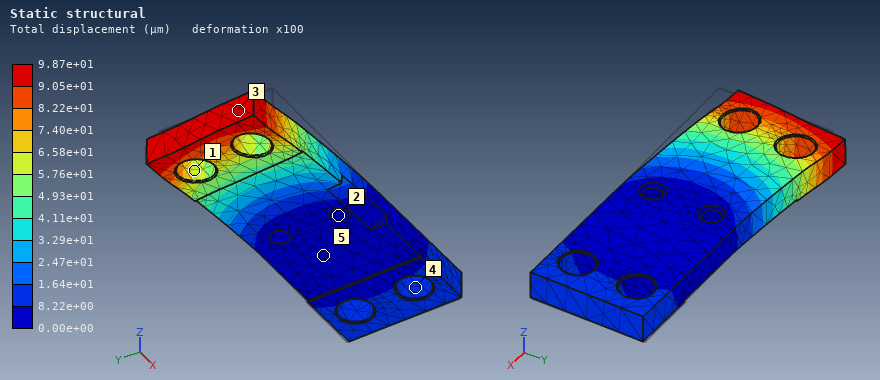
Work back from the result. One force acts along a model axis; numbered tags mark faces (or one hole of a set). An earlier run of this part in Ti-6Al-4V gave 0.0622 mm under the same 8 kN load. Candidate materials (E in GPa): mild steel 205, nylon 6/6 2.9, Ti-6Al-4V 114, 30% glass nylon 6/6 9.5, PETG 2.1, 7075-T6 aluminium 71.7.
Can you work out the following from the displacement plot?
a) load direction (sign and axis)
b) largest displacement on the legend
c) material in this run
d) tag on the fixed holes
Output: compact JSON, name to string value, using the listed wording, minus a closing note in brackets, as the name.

{"load direction": "+Y", "largest displacement on the legend": "9.87e+01 µm", "material in this run": "7075-T6 aluminium", "tag on the fixed holes": "2"}
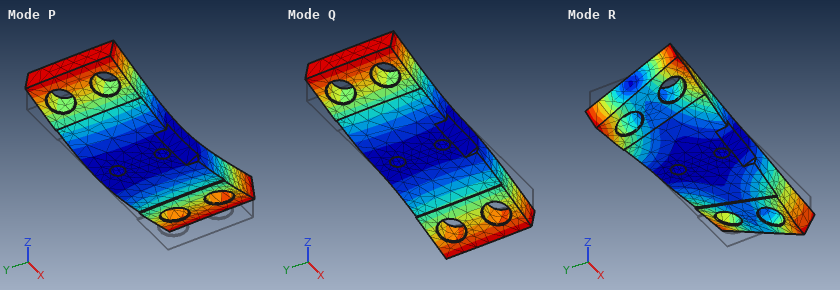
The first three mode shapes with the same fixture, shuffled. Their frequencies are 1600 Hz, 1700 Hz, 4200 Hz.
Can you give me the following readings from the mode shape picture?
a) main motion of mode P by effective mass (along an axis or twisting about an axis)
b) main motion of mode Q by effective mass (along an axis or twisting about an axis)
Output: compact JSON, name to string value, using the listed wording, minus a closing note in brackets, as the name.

{"main motion of mode P by effective mass": "along Z", "main motion of mode Q by effective mass": "twisting about Y"}
